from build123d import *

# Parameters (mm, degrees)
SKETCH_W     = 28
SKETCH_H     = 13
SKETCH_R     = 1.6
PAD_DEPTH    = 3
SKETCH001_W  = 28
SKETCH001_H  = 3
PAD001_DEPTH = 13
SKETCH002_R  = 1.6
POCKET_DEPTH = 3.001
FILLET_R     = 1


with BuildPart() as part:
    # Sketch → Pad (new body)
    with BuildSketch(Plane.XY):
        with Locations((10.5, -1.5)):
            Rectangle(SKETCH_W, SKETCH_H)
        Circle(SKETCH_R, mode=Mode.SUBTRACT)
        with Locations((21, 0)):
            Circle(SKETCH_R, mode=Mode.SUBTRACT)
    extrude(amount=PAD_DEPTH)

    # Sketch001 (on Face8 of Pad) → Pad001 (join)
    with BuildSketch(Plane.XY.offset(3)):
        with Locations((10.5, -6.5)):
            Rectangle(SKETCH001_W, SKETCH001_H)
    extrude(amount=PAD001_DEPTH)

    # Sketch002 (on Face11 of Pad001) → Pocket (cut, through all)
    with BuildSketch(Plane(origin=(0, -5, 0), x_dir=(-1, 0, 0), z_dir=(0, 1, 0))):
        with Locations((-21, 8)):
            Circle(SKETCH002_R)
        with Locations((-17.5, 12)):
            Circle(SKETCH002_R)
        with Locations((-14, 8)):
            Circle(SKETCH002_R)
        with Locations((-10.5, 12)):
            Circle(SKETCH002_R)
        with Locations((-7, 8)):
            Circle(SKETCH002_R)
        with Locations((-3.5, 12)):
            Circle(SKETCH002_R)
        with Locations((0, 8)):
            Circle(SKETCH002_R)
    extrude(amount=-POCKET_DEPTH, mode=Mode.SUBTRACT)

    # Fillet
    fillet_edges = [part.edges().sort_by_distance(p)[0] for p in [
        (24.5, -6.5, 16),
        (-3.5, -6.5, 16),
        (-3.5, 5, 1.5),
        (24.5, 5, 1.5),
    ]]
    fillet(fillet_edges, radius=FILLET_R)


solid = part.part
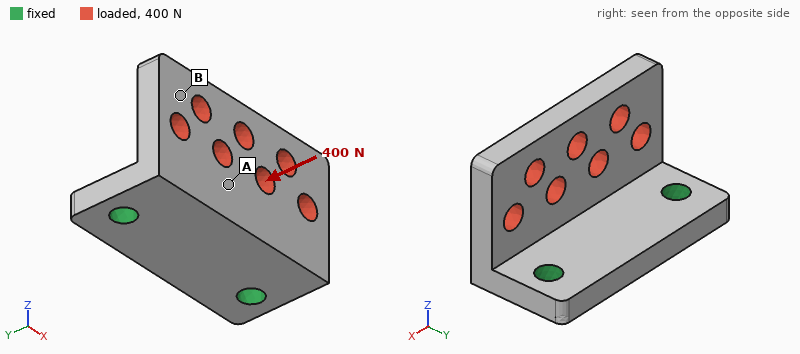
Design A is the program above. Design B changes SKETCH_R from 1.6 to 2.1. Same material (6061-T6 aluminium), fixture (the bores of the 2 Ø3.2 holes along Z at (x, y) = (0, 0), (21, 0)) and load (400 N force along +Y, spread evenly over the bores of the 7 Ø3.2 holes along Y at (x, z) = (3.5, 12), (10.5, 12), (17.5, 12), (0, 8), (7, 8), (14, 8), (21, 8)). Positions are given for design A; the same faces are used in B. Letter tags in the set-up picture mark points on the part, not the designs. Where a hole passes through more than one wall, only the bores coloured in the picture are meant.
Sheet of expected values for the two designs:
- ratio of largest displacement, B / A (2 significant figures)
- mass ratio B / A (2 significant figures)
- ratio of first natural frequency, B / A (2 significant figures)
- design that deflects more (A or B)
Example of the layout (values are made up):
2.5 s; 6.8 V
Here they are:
0.92; 0.98; 1.1; A
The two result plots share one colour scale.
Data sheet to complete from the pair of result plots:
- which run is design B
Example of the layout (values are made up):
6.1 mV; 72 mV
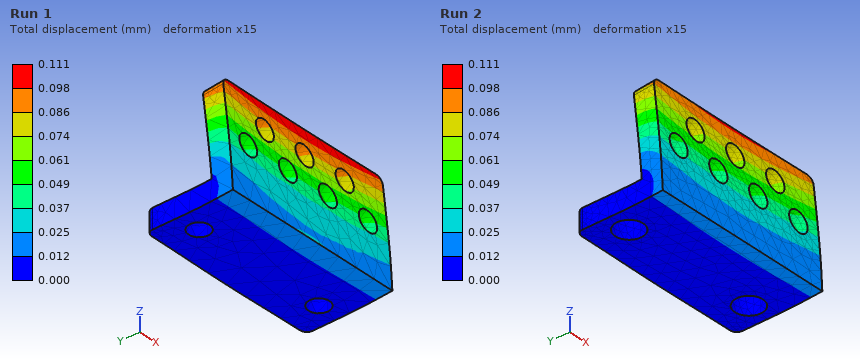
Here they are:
Run 2
